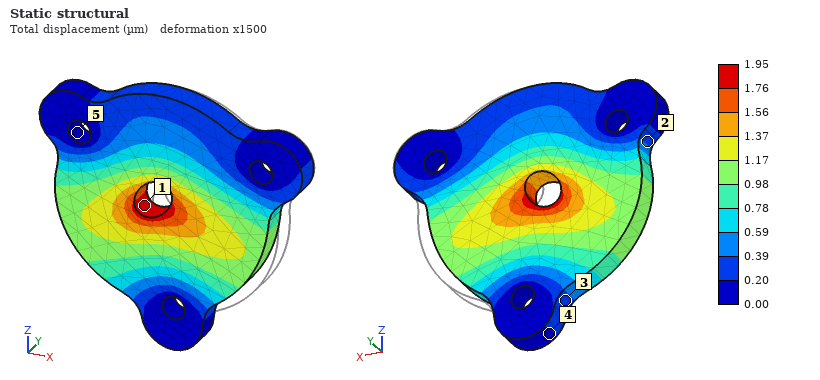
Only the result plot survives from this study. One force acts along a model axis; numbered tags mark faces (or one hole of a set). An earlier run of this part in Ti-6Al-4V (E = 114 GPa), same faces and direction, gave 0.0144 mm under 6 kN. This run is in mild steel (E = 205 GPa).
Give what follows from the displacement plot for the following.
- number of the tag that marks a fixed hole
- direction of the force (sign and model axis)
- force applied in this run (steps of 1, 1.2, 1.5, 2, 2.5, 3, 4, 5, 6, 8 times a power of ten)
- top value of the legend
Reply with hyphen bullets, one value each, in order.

- 5
- -X
- 1.5 kN
- 1.95 µm
